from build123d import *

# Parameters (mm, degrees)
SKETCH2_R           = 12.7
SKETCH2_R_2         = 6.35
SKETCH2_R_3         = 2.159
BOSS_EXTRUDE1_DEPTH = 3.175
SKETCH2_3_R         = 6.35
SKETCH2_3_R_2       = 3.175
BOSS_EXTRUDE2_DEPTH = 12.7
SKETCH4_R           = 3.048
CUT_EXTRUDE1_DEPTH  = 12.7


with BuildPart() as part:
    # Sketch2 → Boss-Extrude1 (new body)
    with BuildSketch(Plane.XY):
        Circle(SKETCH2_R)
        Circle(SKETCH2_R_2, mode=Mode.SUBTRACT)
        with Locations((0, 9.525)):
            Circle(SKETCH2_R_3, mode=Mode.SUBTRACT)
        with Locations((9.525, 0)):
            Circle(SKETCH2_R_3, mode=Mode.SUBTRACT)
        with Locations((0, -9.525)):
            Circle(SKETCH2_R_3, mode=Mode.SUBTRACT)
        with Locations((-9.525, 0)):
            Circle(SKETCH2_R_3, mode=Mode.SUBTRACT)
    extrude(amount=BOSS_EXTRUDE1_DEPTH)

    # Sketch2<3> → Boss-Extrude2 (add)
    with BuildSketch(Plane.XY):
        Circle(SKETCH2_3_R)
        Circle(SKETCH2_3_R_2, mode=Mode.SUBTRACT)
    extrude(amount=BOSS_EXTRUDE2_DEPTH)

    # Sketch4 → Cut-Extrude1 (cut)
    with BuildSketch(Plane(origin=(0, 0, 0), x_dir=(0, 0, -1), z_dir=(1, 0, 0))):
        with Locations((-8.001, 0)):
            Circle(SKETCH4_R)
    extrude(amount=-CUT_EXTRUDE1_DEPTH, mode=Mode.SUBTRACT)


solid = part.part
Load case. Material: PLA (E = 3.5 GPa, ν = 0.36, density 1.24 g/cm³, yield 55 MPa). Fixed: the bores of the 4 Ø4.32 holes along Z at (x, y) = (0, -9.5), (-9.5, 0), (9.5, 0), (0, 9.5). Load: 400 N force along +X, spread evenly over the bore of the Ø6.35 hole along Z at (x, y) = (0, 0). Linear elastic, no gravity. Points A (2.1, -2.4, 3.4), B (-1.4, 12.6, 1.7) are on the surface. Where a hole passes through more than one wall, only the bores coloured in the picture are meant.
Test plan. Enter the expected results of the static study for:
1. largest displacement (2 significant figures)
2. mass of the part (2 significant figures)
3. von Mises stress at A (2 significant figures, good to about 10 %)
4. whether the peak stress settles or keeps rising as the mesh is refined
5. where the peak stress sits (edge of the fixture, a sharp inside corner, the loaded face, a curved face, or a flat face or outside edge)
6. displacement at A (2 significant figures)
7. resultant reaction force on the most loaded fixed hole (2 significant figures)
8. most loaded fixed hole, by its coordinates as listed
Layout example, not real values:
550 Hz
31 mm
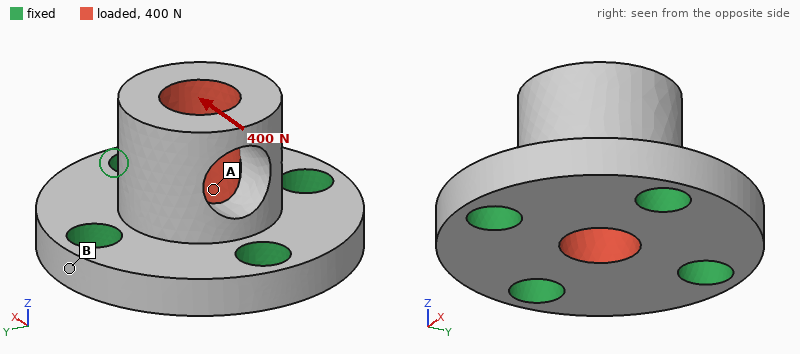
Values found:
65 µm
2.6 g
5.9 MPa
keeps rising
a sharp inside corner
11 µm
190 N
(9.5, 0)
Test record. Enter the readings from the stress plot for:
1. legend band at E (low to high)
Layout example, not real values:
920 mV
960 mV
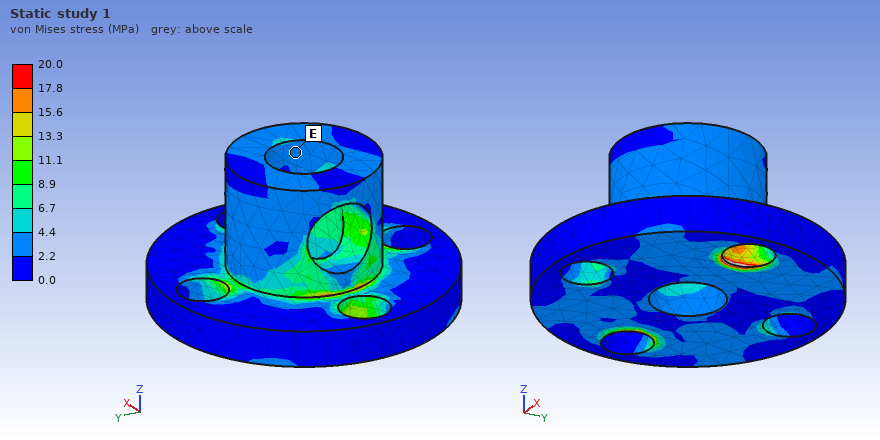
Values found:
2.2 to 4.4 MPa
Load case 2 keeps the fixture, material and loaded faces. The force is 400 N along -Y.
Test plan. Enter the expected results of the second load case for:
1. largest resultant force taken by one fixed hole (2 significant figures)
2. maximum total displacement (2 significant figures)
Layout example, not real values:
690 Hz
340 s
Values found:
170 N
74 µm
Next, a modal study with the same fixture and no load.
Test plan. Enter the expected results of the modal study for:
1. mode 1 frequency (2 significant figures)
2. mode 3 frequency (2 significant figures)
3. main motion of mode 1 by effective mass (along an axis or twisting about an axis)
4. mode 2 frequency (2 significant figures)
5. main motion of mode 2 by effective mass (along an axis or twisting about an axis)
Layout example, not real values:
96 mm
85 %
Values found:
12 kHz
20 kHz
along Y
13 kHz
along X
